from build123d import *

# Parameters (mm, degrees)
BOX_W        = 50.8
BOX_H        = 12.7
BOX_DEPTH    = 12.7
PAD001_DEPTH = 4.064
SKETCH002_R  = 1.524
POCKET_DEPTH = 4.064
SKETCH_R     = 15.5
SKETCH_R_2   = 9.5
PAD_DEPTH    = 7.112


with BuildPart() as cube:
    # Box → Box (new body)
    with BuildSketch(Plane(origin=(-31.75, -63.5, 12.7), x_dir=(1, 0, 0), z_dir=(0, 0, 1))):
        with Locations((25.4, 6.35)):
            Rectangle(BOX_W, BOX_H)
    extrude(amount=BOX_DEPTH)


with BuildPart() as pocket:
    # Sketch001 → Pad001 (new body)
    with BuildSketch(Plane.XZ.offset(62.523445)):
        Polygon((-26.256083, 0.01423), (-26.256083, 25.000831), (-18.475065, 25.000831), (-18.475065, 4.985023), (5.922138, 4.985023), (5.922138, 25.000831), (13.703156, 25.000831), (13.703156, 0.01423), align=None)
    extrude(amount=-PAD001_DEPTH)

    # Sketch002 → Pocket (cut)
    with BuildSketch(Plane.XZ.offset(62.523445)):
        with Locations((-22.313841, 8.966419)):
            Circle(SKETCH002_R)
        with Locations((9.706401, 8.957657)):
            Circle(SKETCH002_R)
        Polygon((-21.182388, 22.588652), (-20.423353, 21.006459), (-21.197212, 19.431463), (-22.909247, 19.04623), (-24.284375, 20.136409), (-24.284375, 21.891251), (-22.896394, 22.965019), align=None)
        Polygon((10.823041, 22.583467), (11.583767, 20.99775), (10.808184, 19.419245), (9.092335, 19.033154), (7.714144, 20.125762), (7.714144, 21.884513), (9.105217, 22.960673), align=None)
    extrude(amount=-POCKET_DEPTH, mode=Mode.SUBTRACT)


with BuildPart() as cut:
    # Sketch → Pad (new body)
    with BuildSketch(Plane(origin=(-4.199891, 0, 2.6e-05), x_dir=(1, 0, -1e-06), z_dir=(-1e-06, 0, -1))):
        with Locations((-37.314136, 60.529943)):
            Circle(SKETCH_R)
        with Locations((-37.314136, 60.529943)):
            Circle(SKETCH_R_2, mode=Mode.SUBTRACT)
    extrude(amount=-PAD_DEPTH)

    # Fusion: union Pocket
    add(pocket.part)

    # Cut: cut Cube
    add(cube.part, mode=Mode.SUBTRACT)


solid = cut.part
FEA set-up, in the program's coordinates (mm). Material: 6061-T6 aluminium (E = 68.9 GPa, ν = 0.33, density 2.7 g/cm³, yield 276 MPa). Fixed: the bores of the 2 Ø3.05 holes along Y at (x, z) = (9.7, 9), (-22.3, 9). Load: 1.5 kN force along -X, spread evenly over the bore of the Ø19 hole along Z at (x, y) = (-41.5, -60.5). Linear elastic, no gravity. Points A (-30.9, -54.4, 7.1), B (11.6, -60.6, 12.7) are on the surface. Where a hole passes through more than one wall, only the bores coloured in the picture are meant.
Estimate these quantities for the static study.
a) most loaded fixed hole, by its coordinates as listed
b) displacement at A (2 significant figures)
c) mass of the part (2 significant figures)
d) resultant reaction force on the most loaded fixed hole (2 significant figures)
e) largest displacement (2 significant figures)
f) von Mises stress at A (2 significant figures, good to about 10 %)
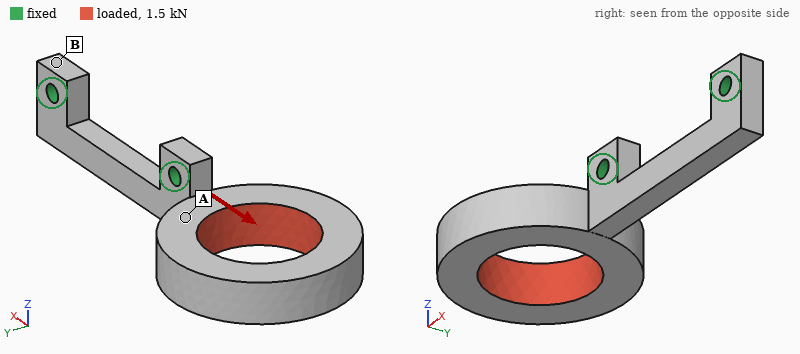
(-22.3, 9)
24 µm
12 g
1.1 kN
100 µm
38 MPa
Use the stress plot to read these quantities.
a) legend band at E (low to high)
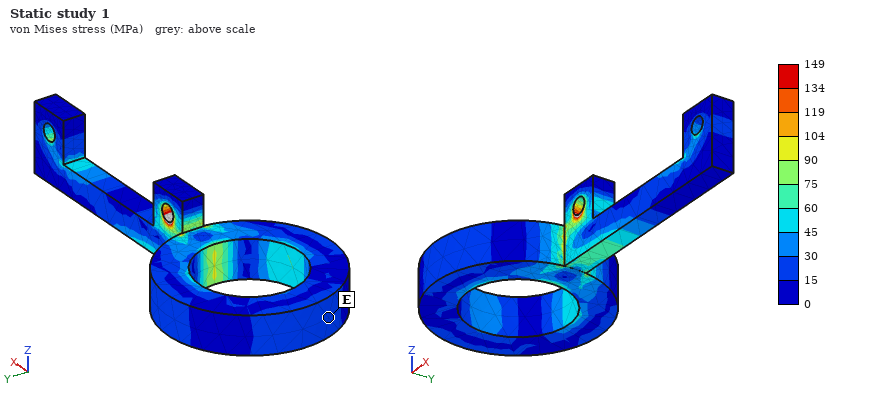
15 to 30 MPa
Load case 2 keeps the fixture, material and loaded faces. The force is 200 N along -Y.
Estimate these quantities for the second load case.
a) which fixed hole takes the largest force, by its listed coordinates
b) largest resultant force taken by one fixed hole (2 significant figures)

(-22.3, 9)
230 N
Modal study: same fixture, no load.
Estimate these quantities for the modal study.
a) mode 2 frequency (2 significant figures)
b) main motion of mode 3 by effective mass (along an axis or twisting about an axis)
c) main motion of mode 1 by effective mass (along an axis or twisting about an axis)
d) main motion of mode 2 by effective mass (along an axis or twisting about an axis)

2400 Hz
twisting about X
along Y
along Z
